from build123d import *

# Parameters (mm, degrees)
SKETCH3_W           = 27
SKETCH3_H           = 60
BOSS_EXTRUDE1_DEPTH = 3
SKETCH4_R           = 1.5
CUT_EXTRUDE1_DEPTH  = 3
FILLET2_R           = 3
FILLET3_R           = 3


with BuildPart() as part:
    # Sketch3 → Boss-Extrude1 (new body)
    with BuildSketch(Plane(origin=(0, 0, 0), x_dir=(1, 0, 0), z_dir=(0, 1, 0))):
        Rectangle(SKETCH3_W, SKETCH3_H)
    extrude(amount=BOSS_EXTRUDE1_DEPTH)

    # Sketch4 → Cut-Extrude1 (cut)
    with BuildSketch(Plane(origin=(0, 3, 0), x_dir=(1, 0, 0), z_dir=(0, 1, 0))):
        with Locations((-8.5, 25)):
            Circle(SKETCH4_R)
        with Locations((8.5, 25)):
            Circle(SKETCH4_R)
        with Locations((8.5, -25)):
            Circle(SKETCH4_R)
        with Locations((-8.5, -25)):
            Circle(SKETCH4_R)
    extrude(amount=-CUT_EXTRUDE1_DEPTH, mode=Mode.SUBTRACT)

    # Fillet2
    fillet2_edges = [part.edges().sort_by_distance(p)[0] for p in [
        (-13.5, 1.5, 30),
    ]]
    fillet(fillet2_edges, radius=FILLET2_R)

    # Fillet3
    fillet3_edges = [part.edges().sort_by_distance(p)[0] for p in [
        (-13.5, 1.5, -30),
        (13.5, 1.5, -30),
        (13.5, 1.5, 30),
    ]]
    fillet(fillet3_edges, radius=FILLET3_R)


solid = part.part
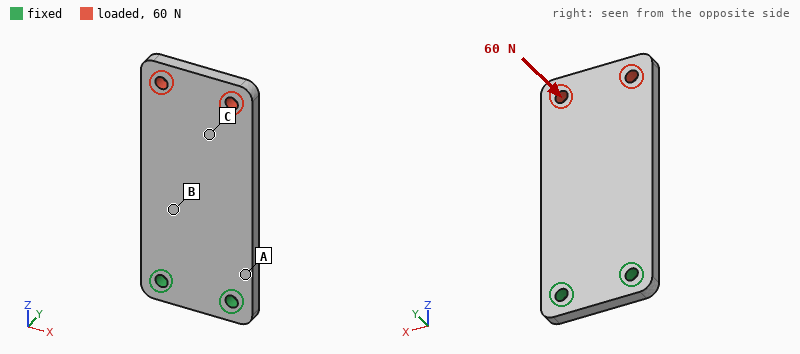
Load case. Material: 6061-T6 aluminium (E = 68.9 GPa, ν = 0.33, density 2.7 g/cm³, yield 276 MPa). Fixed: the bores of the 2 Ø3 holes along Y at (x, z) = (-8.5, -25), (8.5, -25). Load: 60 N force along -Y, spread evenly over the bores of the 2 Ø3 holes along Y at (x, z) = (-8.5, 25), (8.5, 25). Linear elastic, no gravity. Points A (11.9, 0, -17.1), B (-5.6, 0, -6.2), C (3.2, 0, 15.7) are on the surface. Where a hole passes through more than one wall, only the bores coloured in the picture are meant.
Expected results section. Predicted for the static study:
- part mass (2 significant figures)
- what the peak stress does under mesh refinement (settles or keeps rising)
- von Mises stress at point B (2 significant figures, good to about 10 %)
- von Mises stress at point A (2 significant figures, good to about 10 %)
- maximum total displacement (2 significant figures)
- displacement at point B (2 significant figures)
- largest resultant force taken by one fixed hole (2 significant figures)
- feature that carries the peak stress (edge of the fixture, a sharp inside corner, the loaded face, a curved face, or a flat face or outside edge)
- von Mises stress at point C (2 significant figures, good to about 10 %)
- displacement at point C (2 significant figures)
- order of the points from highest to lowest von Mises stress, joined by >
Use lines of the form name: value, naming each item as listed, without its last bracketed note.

part mass: 13 g
what the peak stress does under mesh refinement: keeps rising
von Mises stress at point B: 45 MPa
von Mises stress at point A: 65 MPa
maximum total displacement: 0.68 mm
displacement at point B: 0.11 mm
largest resultant force taken by one fixed hole: 30 N
feature that carries the peak stress: edge of the fixture
von Mises stress at point C: 14 MPa
displacement at point C: 0.43 mm
order of the points from highest to lowest von Mises stress, joined by >: A > B > C
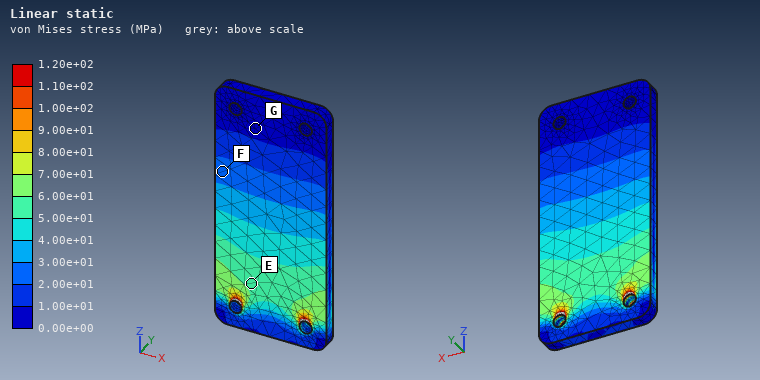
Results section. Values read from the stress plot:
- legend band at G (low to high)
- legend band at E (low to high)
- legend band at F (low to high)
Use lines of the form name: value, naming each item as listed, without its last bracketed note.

legend band at G: 0.00e+00 to 1.00e+01 MPa
legend band at E: 5.00e+01 to 6.00e+01 MPa
legend band at F: 2.00e+01 to 3.00e+01 MPa
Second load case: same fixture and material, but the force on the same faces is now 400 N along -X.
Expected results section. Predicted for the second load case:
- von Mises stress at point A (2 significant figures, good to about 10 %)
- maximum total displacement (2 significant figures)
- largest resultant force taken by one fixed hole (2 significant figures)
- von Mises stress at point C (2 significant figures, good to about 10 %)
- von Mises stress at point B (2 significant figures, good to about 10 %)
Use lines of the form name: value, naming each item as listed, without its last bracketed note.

von Mises stress at point A: 38 MPa
maximum total displacement: 75 µm
largest resultant force taken by one fixed hole: 1.1 kN
von Mises stress at point C: 12 MPa
von Mises stress at point B: 18 MPa
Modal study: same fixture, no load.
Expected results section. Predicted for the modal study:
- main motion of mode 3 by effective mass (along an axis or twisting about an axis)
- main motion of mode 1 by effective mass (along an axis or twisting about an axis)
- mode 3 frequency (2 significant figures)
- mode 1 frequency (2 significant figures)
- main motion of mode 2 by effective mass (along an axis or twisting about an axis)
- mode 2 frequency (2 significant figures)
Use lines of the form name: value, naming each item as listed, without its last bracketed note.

main motion of mode 3 by effective mass: along Y
main motion of mode 1 by effective mass: along Y
mode 3 frequency: 5100 Hz
mode 1 frequency: 830 Hz
main motion of mode 2 by effective mass: twisting about Z
mode 2 frequency: 3500 Hz
